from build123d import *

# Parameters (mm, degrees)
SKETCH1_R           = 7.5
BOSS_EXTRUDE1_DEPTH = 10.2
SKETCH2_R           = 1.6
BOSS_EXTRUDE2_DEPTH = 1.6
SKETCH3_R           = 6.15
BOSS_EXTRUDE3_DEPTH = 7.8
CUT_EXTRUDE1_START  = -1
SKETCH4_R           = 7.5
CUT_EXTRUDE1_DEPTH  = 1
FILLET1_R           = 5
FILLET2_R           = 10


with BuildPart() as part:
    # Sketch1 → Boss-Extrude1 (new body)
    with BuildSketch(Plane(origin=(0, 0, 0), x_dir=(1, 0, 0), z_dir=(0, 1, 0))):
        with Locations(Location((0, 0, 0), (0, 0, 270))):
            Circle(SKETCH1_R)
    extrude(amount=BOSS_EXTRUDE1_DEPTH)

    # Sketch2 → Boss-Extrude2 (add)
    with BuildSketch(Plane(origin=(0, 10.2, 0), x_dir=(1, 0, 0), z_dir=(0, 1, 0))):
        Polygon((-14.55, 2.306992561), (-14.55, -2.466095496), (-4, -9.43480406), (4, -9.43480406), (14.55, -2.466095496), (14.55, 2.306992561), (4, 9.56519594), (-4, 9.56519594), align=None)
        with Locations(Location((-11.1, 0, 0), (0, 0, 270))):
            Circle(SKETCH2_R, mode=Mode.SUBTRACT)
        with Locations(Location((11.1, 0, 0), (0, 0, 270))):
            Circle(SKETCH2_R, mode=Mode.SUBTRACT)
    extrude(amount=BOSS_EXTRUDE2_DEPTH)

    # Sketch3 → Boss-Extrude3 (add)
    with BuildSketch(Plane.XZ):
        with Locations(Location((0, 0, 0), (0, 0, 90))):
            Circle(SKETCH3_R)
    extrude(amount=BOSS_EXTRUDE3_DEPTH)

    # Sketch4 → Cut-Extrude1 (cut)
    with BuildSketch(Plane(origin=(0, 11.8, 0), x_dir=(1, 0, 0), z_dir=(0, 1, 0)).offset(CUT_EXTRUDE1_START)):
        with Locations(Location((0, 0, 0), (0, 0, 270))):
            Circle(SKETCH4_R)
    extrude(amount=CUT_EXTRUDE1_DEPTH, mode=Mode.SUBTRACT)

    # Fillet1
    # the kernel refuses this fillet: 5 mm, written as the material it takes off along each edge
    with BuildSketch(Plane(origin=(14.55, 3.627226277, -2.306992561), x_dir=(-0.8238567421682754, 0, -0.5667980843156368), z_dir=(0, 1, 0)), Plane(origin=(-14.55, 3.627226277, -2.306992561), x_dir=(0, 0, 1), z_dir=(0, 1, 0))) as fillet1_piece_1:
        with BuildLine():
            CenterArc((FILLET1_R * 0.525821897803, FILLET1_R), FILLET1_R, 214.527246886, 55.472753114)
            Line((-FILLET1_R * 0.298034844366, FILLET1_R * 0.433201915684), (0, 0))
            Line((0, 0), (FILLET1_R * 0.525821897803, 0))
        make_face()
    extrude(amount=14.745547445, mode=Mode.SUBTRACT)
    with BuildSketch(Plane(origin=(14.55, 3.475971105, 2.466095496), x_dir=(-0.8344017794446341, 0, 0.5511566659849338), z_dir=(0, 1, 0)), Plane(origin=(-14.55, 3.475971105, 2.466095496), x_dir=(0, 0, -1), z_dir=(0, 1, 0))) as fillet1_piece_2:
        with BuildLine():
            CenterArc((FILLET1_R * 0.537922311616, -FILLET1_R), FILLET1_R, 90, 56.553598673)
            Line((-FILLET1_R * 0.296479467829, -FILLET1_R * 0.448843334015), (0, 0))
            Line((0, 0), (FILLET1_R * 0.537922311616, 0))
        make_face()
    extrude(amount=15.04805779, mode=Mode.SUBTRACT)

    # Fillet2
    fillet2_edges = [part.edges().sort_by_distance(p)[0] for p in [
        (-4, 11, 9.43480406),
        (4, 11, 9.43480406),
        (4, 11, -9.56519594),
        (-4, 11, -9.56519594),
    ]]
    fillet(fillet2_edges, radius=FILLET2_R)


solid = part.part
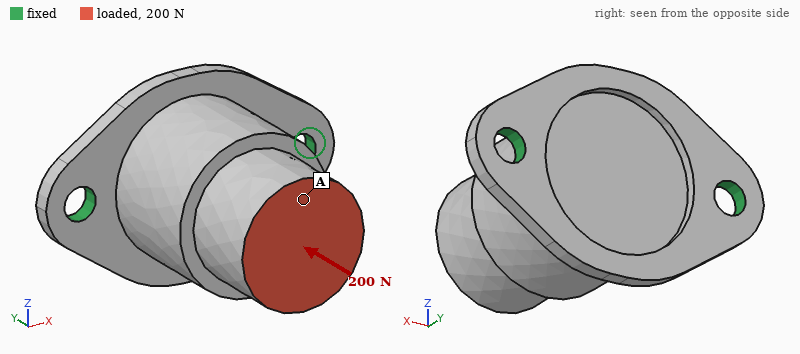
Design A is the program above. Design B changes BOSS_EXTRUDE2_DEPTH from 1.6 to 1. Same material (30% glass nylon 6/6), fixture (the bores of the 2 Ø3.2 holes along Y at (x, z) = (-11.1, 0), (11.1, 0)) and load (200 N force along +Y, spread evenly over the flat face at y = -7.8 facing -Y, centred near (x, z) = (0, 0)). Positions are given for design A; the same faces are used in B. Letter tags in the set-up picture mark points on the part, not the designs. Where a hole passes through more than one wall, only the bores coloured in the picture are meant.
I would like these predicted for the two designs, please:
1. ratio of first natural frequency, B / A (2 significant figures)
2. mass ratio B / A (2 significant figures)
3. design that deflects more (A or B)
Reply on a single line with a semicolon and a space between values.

0.61; 0.96; B
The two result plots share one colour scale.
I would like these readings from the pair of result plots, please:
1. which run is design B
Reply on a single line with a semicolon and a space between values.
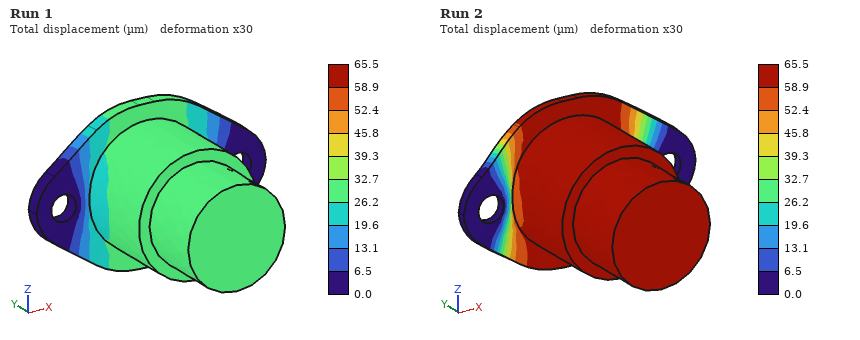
Run 2
